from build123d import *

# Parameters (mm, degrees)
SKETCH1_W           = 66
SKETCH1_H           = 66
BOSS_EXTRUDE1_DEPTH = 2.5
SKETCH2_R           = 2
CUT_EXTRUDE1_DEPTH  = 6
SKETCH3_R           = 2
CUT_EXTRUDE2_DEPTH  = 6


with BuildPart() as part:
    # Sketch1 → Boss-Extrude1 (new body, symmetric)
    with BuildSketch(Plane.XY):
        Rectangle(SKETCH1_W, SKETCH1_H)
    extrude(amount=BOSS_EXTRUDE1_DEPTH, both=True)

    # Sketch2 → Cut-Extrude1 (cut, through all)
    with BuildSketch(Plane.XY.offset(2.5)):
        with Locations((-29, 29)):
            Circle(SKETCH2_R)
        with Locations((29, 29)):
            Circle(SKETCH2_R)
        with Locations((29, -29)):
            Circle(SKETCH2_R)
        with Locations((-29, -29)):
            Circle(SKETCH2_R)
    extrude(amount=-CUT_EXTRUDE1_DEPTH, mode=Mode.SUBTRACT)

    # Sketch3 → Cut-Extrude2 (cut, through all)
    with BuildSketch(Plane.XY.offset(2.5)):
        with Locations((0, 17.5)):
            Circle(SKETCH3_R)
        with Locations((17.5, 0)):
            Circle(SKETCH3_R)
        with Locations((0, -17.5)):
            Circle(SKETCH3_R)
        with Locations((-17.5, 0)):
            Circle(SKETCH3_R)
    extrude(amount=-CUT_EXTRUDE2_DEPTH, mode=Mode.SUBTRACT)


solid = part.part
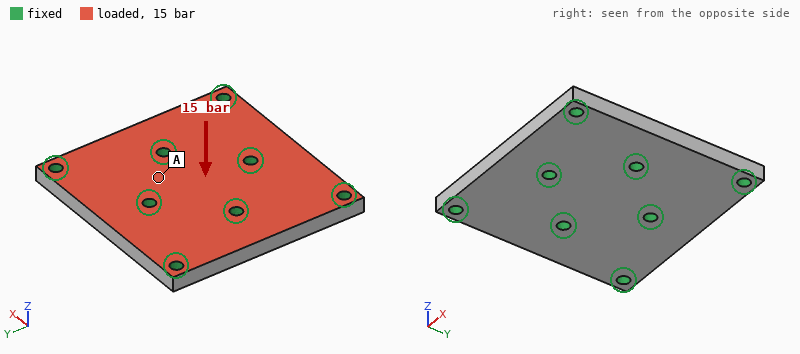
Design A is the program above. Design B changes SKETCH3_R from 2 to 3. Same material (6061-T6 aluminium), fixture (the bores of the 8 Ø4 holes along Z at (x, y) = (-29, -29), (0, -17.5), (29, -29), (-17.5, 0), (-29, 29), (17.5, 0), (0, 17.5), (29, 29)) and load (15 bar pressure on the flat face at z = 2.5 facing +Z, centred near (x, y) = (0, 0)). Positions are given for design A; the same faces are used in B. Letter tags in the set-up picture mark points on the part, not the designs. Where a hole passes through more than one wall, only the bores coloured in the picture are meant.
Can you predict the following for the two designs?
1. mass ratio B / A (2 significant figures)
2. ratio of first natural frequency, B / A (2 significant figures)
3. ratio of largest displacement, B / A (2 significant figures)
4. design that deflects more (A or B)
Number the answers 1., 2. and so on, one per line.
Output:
1. 0.99
2. 1.1
3. 0.81
4. A
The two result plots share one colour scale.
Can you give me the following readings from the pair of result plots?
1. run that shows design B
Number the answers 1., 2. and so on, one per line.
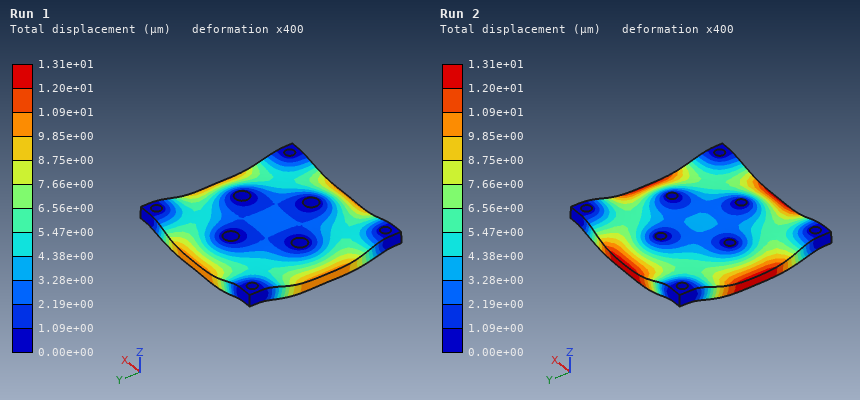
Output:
1. Run 1
